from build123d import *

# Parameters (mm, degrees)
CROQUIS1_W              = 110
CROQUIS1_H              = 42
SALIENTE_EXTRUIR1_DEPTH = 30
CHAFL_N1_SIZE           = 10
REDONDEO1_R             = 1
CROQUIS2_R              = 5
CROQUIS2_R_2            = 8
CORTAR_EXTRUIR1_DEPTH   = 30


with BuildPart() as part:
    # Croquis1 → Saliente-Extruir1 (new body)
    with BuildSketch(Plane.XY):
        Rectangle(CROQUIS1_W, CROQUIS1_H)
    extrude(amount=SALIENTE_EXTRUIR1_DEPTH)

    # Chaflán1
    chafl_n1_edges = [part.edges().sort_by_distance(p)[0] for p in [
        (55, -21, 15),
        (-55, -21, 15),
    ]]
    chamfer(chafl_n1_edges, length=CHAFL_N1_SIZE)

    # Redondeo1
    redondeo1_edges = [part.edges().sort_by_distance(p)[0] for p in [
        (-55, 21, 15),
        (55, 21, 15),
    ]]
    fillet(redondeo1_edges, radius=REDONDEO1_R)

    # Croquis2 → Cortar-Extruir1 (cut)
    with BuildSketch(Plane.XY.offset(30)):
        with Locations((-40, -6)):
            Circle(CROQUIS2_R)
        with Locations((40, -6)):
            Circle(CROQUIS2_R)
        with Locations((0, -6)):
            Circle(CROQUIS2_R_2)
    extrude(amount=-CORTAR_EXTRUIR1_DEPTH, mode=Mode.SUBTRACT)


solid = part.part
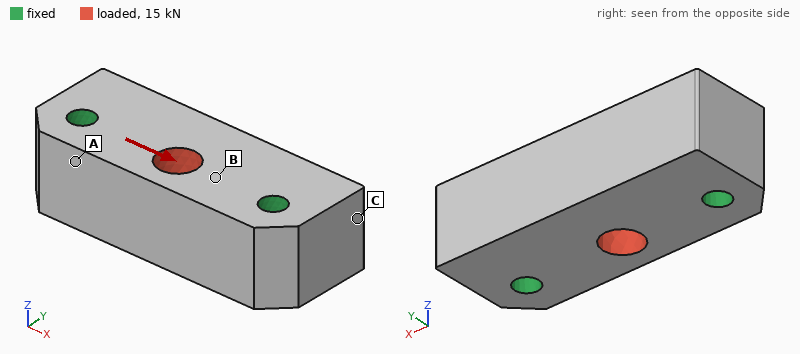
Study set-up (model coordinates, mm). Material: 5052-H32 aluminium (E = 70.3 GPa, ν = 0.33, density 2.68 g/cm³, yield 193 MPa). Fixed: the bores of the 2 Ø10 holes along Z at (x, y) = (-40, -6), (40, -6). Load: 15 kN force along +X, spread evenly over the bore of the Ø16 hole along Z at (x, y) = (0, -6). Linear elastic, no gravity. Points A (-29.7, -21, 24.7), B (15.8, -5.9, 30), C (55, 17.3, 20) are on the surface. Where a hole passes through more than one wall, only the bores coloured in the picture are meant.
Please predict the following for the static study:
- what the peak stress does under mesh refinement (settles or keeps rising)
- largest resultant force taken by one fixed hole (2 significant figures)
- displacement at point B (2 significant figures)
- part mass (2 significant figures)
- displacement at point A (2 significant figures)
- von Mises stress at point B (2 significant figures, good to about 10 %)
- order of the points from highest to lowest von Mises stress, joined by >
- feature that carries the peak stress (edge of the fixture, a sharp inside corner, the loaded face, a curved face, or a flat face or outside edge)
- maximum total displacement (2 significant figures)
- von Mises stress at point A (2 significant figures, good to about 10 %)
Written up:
keeps rising
7.5 kN
3.2 µm
330 g
1.8 µm
11 MPa
B > A > C
edge of the fixture
5.1 µm
5.1 MPa
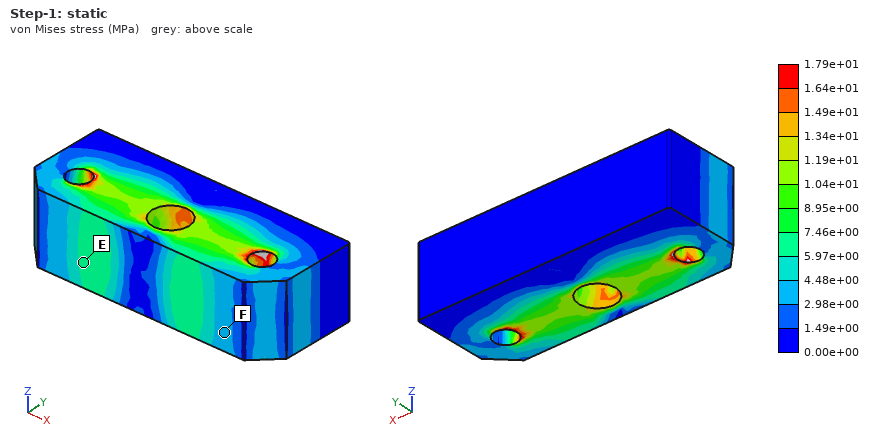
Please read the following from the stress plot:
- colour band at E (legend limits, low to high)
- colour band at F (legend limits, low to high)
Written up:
5.97e+00 to 7.46e+00 MPa
2.98e+00 to 4.48e+00 MPa
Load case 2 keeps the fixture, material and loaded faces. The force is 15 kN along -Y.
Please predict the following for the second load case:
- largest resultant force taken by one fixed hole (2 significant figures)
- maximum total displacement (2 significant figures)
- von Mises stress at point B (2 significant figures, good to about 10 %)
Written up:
7.9 kN
19 µm
15 MPa
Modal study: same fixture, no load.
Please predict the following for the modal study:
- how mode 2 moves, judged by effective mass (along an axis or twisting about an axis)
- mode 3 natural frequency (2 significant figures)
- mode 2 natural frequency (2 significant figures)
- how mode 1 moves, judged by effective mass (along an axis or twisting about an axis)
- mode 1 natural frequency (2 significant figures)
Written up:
along Y
17 kHz
14 kHz
along Z
13 kHz
